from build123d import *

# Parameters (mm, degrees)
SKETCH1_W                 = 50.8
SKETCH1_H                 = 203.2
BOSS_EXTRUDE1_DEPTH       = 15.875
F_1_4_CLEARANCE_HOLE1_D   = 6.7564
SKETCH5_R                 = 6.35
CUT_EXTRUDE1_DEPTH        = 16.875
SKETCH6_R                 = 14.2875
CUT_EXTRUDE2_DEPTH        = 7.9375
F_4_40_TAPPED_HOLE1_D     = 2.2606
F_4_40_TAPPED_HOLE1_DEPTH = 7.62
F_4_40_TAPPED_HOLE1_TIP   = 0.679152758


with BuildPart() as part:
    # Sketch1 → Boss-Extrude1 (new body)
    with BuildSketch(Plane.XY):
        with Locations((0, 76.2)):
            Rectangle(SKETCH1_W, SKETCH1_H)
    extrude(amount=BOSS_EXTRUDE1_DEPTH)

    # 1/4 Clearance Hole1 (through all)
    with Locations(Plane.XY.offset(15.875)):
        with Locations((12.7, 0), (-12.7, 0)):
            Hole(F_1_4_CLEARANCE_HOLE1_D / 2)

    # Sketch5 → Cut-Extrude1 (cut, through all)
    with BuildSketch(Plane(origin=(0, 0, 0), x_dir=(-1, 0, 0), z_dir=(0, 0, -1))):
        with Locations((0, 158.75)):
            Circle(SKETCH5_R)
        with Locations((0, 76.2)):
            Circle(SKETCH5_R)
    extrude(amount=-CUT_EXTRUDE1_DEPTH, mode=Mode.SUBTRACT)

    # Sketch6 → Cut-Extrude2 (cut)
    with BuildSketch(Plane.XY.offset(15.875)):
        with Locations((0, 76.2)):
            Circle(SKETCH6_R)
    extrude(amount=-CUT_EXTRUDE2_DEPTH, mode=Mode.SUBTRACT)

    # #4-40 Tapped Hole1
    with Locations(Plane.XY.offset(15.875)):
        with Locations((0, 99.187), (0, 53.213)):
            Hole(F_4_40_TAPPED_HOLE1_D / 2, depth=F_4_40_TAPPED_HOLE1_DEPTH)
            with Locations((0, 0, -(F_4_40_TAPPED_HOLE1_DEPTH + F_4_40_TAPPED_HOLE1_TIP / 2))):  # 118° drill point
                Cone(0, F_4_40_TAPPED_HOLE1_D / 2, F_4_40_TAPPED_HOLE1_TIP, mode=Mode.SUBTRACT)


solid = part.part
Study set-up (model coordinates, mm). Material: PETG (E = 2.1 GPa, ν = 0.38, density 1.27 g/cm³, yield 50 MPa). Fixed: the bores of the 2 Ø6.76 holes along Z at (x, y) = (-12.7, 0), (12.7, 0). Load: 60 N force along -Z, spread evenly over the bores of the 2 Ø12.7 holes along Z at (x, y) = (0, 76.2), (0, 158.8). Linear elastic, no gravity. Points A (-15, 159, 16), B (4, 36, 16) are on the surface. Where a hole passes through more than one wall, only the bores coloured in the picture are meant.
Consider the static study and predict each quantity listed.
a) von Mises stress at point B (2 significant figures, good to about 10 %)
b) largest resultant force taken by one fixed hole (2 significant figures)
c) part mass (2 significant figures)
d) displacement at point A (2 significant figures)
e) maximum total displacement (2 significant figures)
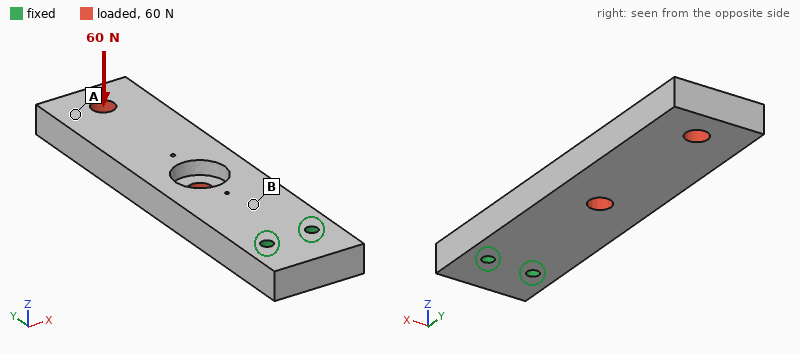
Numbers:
2.5 MPa
30 N
200 g
1.9 mm
2.2 mm
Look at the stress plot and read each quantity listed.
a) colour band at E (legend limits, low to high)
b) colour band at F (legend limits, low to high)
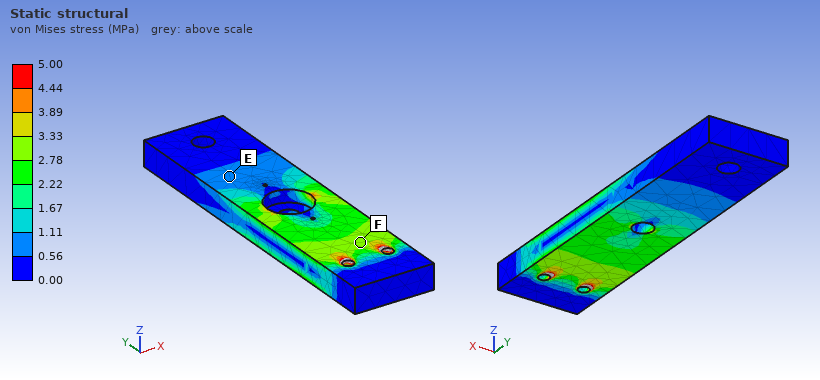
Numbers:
0.56 to 1.11 MPa
2.78 to 3.33 MPa
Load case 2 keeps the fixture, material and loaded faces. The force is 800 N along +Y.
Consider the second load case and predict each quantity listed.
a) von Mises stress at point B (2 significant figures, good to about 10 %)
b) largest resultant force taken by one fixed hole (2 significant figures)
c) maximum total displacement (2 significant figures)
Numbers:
0.46 MPa
400 N
0.23 mm
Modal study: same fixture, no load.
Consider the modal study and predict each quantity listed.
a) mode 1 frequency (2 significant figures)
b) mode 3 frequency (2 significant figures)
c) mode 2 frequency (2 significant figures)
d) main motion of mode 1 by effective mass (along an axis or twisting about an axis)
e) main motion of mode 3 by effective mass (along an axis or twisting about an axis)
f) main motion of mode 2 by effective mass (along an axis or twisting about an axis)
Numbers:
100 Hz
570 Hz
300 Hz
along Z
twisting about Y
along X
